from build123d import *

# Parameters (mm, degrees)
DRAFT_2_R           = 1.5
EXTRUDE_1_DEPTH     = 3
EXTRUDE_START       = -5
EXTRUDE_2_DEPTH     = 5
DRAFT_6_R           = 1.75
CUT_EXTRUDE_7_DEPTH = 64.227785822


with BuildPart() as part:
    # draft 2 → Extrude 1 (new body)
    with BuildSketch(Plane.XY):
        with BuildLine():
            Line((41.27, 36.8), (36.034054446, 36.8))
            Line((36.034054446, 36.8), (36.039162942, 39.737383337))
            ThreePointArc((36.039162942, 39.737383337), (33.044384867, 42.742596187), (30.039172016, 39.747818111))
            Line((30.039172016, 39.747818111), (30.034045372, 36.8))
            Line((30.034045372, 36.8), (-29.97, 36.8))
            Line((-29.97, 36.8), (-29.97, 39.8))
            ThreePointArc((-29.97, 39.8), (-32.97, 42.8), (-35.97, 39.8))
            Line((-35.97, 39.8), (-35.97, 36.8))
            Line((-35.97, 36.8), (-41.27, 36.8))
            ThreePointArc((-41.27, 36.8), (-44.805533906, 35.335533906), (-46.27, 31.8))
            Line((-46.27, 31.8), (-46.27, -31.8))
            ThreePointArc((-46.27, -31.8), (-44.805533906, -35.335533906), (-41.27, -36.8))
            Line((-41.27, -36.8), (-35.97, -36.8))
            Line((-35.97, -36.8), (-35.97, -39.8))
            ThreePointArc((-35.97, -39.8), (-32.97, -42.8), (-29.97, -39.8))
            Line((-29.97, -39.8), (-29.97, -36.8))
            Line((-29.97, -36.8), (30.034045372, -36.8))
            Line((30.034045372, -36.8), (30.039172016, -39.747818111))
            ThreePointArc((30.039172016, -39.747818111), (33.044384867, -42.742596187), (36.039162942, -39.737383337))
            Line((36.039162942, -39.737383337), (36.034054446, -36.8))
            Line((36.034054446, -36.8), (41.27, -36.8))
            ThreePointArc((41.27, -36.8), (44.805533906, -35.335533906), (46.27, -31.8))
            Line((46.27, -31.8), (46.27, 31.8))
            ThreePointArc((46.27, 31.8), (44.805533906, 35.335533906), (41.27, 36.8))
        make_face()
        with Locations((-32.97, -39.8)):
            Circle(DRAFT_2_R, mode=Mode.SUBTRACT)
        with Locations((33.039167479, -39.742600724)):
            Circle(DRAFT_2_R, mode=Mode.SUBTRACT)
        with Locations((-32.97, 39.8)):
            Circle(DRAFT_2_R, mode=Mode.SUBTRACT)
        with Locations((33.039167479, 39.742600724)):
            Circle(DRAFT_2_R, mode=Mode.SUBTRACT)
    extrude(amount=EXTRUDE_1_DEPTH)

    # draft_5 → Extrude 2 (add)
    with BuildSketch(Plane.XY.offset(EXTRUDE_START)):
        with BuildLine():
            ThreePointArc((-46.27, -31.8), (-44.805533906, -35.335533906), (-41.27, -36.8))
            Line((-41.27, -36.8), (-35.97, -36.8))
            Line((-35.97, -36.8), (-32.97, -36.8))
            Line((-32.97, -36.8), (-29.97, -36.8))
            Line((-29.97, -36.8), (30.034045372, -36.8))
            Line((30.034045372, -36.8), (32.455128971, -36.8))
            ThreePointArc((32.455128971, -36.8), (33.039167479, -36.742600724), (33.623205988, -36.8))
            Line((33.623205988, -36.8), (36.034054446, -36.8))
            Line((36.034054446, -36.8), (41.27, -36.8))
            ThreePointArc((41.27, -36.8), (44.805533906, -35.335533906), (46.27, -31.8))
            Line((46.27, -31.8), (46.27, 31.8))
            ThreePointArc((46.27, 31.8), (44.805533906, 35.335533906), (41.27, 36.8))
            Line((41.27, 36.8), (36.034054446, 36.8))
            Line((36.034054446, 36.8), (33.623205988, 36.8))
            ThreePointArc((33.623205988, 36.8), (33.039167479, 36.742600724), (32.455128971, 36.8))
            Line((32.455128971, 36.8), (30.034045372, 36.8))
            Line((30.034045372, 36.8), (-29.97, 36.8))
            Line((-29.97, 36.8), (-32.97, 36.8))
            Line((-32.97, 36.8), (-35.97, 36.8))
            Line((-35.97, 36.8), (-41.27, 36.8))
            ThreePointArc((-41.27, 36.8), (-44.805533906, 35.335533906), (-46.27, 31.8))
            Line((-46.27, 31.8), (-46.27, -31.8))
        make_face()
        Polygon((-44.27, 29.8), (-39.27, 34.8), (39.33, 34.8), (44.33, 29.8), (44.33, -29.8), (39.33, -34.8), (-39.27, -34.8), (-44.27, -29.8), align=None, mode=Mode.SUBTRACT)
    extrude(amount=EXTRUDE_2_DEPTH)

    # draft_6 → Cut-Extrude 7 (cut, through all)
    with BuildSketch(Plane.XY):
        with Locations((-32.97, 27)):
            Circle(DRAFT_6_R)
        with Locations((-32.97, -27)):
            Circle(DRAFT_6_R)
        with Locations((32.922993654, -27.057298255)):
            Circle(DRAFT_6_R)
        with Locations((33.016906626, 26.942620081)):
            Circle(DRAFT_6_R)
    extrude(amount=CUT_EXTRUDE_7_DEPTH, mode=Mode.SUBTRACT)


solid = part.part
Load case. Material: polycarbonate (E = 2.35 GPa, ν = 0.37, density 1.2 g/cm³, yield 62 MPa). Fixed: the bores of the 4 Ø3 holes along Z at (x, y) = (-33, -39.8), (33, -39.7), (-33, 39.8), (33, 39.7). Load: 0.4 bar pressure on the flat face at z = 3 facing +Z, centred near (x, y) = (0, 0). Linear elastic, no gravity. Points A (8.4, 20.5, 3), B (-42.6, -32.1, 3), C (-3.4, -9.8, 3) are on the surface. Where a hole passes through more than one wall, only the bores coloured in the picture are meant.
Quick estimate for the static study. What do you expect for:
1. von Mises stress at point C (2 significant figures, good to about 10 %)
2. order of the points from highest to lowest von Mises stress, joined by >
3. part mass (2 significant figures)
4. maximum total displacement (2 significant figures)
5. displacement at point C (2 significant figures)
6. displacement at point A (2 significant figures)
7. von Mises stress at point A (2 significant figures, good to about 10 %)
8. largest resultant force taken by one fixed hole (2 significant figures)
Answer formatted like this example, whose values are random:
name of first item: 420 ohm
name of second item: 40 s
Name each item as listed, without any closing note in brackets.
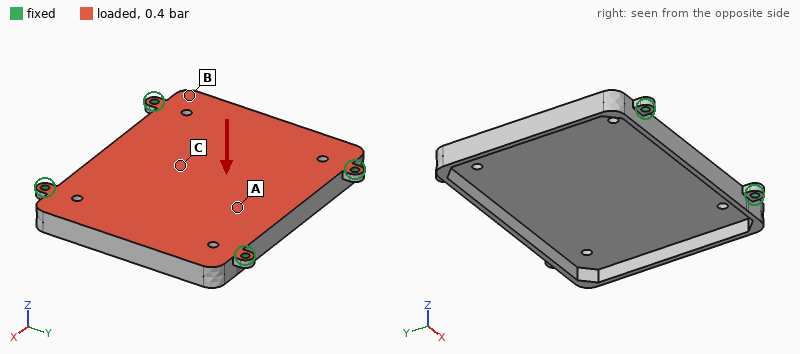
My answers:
von Mises stress at point C: 8.3 MPa
order of the points from highest to lowest von Mises stress, joined by >: C > A > B
part mass: 29 g
maximum total displacement: 1.4 mm
displacement at point C: 1.3 mm
displacement at point A: 0.95 mm
von Mises stress at point A: 6.1 MPa
largest resultant force taken by one fixed hole: 72 N
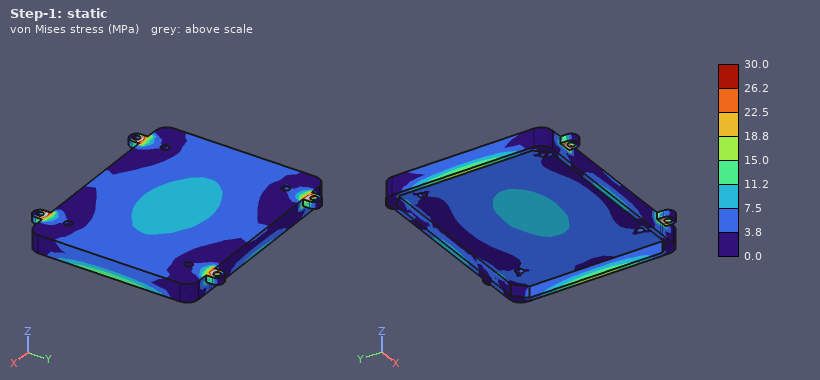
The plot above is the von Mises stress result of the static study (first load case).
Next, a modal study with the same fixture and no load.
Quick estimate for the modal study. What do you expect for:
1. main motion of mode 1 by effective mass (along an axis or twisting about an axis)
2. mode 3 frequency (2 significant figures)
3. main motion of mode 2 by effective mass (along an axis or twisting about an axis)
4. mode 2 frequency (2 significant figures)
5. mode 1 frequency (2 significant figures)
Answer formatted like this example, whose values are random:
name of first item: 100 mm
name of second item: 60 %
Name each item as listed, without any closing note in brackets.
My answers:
main motion of mode 1 by effective mass: along Z
mode 3 frequency: 900 Hz
main motion of mode 2 by effective mass: twisting about Y
mode 2 frequency: 790 Hz
mode 1 frequency: 550 Hz
